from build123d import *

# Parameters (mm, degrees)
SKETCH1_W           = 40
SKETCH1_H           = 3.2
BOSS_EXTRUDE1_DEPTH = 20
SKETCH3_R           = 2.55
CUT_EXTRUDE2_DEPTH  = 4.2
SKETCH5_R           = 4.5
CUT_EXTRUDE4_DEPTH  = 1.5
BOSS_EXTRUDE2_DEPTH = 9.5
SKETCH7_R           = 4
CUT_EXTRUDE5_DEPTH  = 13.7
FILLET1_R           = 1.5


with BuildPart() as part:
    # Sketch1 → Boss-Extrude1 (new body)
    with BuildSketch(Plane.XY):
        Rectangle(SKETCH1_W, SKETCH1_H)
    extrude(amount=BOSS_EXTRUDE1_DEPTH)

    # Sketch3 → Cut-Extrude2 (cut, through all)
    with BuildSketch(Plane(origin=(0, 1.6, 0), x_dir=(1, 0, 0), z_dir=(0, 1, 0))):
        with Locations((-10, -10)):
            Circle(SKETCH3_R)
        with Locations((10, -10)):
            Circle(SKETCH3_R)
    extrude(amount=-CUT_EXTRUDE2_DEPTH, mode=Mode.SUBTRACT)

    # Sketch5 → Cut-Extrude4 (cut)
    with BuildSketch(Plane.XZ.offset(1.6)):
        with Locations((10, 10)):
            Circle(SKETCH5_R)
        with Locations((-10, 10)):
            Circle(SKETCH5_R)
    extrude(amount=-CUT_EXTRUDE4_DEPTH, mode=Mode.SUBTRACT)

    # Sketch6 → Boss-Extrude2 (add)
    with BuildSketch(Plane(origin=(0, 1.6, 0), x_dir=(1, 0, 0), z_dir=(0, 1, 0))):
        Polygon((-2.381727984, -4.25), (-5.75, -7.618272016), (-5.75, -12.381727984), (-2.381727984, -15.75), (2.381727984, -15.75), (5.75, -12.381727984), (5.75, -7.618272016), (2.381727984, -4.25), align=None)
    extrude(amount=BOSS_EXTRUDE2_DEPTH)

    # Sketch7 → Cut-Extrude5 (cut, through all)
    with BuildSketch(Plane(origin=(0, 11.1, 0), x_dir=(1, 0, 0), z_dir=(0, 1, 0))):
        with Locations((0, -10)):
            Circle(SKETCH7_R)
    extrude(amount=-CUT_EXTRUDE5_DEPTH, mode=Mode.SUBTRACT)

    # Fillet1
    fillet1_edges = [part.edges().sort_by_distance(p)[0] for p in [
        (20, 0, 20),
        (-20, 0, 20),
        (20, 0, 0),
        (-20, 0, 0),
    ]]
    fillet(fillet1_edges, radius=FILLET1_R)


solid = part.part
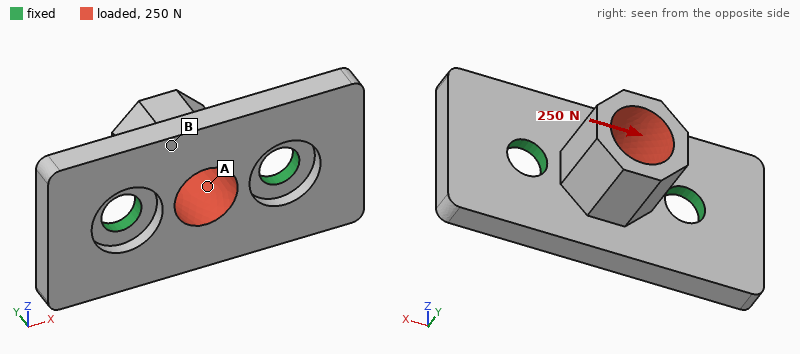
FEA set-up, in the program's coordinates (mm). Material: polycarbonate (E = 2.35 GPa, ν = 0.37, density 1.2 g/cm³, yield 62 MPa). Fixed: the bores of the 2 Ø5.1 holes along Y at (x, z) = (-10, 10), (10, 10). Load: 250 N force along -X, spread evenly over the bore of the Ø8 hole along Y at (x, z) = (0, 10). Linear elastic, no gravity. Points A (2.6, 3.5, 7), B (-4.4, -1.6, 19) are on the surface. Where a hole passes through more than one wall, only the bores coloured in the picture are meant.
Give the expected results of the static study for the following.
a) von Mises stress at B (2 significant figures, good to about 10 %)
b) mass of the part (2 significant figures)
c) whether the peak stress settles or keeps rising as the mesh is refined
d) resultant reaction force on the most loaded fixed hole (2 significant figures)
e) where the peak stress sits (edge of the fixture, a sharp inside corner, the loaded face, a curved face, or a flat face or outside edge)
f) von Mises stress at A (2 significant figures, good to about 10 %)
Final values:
2.8 MPa
3.2 g
keeps rising
140 N
edge of the fixture
7.8 MPa
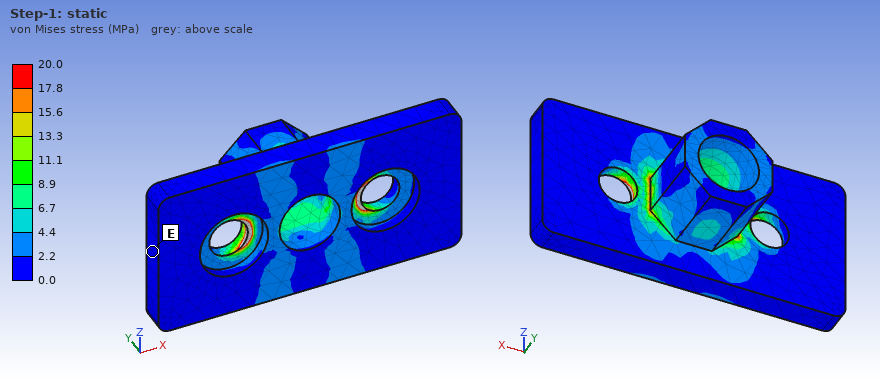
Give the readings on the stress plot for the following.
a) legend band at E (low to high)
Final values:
0.0 to 2.2 MPa
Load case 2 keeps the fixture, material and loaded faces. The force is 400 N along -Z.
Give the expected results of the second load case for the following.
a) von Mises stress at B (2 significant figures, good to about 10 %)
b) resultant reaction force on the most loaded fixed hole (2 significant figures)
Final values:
11 MPa
200 N
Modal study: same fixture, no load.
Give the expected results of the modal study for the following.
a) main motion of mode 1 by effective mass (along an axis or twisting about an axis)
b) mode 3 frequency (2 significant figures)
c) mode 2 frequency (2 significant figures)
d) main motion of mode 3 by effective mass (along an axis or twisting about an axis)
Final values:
twisting about X
5000 Hz
4800 Hz
twisting about Z
